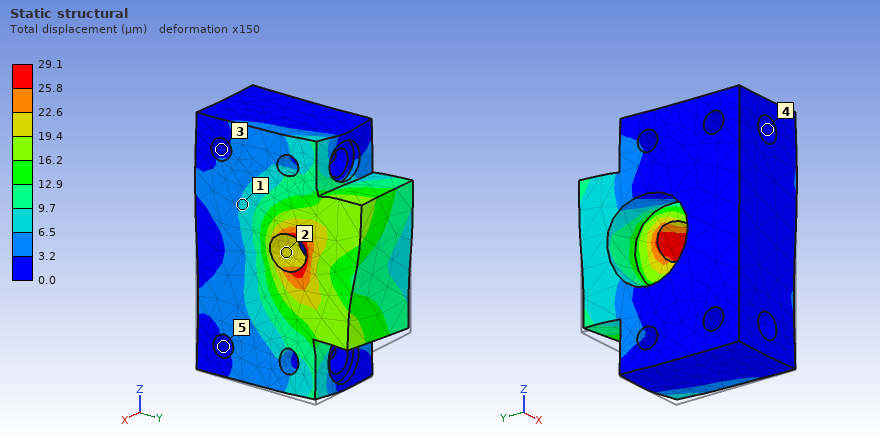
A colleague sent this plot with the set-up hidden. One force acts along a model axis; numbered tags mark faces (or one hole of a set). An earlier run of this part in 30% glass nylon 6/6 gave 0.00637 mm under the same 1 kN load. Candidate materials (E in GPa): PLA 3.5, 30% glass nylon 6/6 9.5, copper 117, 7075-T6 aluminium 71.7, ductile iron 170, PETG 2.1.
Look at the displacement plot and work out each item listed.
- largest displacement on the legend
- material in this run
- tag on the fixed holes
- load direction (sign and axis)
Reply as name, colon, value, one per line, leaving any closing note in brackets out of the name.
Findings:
largest displacement on the legend: 29.1 µm
material in this run: PETG
tag on the fixed holes: 4
load direction: +Z
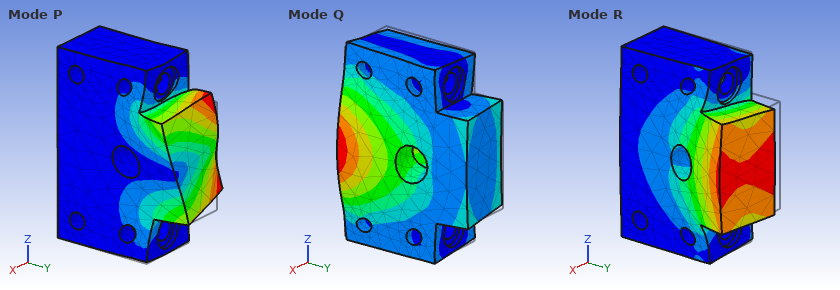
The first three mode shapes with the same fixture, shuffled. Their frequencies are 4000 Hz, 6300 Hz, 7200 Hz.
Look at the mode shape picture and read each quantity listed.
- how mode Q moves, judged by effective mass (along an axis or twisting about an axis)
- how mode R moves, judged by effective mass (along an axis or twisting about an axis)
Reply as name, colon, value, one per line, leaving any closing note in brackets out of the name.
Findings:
how mode Q moves, judged by effective mass: along X
how mode R moves, judged by effective mass: along X
